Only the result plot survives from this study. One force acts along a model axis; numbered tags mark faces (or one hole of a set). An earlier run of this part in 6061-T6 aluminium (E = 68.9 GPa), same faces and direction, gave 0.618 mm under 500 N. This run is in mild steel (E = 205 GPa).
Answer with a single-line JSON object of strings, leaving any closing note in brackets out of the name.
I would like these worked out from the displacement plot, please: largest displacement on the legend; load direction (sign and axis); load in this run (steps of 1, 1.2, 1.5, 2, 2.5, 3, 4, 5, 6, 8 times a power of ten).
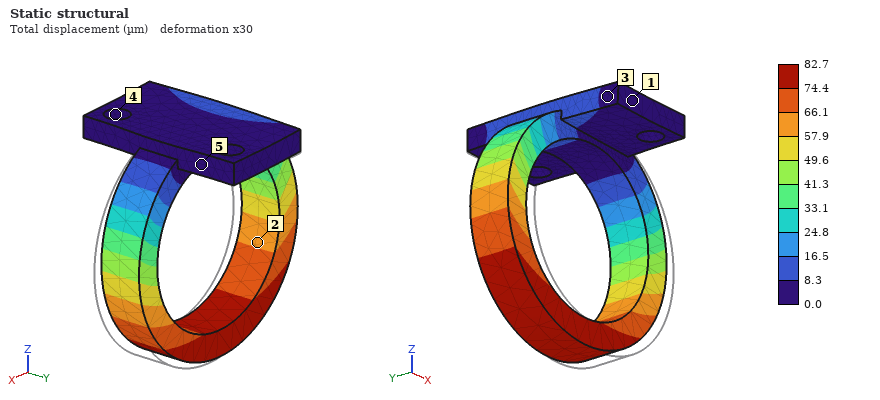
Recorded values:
{"largest displacement on the legend": "82.7 µm", "load direction": "-X", "load in this run": "200 N"}
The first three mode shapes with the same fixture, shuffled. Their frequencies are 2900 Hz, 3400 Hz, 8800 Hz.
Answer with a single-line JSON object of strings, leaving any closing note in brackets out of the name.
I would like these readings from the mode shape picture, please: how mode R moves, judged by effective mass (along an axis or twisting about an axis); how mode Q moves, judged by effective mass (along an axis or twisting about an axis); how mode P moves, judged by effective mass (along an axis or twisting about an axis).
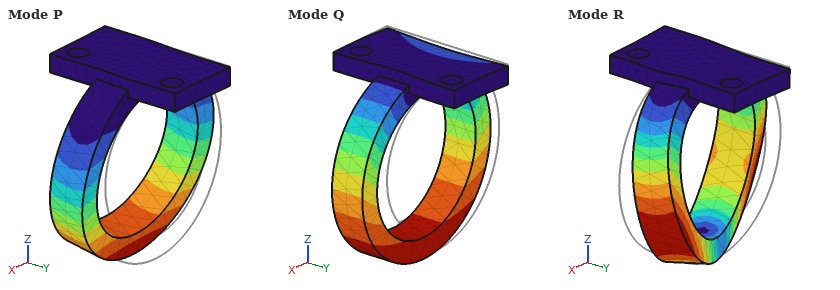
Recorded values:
{"how mode R moves, judged by effective mass": "twisting about Z", "how mode Q moves, judged by effective mass": "along X", "how mode P moves, judged by effective mass": "along Y"}
